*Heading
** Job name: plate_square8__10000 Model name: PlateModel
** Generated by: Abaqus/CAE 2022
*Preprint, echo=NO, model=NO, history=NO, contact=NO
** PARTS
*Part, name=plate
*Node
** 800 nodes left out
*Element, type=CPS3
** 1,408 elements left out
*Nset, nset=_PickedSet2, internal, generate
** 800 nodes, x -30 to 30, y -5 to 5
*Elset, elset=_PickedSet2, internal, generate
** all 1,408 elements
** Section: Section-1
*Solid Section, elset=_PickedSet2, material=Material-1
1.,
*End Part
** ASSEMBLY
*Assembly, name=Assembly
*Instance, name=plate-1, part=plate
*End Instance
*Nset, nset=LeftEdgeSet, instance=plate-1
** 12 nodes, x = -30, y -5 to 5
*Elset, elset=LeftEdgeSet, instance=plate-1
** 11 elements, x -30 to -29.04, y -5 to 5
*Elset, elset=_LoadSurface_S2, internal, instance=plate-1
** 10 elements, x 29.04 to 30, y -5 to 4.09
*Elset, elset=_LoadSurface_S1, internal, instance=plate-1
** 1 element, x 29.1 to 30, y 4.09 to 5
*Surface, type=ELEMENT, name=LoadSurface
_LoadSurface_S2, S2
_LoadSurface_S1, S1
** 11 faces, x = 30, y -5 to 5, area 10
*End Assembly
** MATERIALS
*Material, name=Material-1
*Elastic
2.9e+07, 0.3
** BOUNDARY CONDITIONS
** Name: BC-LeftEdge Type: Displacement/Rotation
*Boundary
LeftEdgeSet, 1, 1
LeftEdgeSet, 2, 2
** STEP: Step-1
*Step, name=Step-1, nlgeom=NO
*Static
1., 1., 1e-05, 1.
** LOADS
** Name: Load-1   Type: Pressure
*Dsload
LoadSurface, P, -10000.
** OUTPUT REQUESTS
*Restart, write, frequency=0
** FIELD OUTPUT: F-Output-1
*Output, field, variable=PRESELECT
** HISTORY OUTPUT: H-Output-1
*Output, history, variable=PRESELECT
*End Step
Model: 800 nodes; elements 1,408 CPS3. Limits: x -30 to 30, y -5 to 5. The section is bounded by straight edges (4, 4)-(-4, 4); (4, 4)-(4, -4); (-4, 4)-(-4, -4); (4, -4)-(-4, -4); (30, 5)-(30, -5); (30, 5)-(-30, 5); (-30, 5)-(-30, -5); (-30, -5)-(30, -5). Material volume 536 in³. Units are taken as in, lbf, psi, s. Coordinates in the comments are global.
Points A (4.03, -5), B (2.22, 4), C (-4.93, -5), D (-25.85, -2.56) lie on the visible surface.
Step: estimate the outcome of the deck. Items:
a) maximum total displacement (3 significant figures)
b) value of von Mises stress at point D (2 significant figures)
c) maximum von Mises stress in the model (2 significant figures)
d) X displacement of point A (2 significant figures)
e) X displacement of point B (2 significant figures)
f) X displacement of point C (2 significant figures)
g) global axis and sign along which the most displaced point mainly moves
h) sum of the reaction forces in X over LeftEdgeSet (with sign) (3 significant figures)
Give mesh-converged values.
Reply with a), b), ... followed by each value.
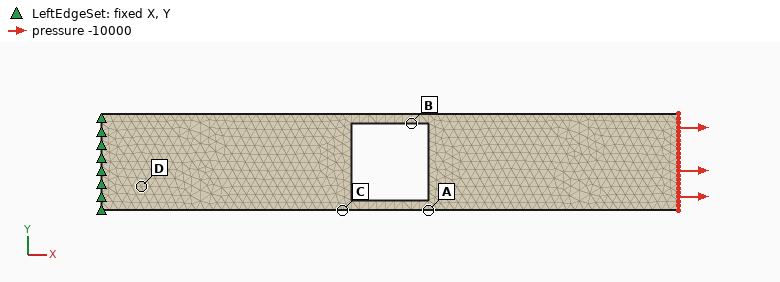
a) 0.0385 in
b) 10000 psi
c) 60000 psi
d) 0.025 in
e) 0.024 in
f) 0.012 in
g) +X
h) -1.00e+05 lbf
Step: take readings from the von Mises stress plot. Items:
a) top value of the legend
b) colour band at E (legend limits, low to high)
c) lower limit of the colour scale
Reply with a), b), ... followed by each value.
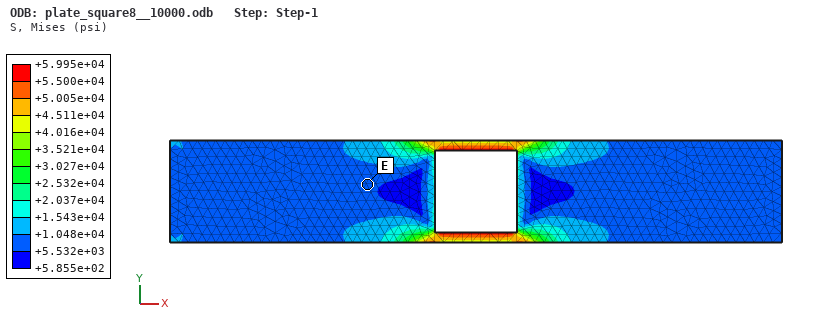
a) +5.995e+04 psi
b) +5.532e+03 to +1.048e+04 psi
c) +5.855e+02 psi
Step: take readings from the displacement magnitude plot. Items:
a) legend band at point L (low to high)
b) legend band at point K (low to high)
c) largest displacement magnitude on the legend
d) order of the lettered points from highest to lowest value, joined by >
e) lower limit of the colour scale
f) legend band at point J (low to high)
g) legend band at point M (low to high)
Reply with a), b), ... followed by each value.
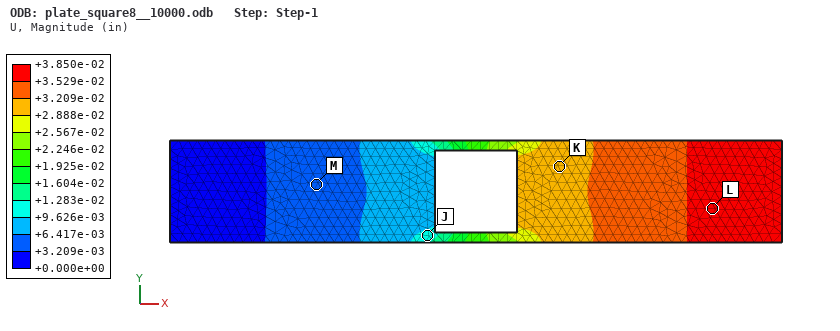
a) +3.529e-02 to +3.850e-02 in
b) +2.888e-02 to +3.209e-02 in
c) +3.850e-02 in
d) L > K > J > M
e) +0.000e+00 in
f) +9.626e-03 to +1.283e-02 in
g) +3.209e-03 to +6.417e-03 in
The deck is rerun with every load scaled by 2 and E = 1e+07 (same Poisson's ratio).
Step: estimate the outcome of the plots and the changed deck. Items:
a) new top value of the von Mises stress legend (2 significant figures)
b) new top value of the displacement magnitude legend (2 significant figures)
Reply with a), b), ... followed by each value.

a) 1.2e+05 psi
b) 0.22 in
